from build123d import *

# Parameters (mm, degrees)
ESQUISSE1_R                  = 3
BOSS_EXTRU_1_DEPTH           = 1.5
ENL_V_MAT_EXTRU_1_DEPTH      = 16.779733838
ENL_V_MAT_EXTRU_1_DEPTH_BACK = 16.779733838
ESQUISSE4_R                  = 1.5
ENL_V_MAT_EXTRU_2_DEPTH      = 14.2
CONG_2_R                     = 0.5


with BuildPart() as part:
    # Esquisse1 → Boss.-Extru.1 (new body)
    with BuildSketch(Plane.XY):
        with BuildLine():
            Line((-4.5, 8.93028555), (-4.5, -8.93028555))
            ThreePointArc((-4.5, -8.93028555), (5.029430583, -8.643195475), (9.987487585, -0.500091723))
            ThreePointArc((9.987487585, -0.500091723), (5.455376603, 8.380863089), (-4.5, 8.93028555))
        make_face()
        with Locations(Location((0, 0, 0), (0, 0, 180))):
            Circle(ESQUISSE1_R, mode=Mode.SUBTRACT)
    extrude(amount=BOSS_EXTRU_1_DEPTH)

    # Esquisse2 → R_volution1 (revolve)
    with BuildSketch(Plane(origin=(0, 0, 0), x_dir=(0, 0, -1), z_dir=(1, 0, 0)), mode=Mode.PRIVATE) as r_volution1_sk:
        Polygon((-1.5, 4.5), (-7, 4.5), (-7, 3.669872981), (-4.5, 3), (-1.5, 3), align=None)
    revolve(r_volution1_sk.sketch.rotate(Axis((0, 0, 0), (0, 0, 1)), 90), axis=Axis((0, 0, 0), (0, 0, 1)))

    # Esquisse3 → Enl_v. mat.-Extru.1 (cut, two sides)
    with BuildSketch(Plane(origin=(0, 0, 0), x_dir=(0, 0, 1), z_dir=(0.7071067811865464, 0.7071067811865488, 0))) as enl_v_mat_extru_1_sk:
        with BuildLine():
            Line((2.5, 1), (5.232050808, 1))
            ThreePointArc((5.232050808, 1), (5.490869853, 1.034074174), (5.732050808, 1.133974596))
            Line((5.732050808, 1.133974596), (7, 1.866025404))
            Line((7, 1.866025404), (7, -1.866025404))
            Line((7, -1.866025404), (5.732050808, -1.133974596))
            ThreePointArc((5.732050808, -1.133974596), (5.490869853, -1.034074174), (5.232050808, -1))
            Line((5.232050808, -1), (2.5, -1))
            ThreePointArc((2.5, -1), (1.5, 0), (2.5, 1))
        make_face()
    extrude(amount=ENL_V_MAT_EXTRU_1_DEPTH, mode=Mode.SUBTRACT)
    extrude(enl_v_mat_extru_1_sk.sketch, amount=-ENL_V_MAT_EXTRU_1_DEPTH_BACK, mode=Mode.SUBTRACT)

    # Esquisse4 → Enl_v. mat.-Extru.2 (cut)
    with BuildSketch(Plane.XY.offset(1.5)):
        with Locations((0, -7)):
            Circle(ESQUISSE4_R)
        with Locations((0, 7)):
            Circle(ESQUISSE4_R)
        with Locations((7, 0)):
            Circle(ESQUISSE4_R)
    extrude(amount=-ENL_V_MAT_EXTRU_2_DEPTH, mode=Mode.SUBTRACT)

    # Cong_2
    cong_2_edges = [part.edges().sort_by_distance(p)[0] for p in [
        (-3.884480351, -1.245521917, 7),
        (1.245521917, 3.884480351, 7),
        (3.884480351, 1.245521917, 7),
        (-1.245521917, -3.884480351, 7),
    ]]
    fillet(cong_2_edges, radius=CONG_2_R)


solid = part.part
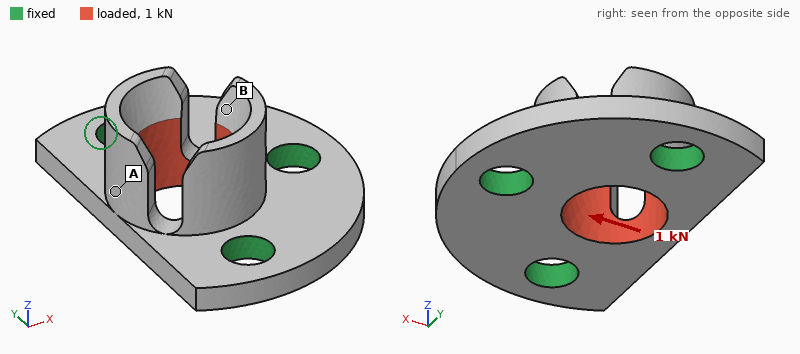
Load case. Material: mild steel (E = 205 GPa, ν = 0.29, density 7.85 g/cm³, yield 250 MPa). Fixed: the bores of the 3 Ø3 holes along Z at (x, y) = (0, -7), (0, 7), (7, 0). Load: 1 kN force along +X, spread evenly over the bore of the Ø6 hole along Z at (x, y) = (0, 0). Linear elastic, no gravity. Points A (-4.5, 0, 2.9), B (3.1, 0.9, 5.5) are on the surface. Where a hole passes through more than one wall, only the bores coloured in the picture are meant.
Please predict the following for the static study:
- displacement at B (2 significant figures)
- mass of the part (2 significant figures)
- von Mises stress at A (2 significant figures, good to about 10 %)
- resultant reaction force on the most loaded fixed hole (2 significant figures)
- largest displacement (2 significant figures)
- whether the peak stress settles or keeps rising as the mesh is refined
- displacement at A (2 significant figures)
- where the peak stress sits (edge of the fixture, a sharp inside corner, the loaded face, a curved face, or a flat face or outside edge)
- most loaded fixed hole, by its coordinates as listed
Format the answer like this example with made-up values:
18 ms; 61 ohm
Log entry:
4.4 µm; 3.4 g; 53 MPa; 410 N; 15 µm; keeps rising; 8.8 µm; edge of the fixture; (7, 0)
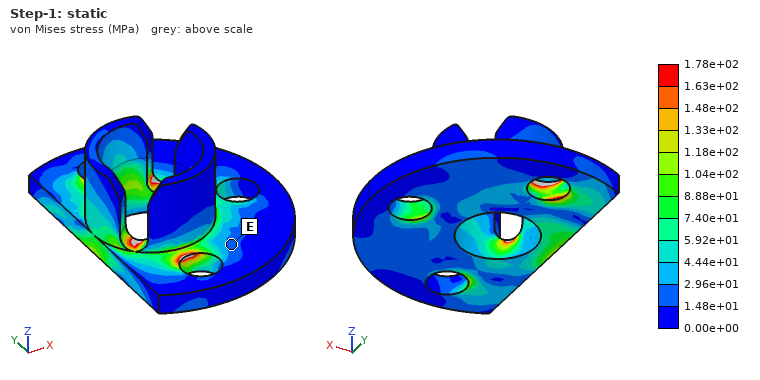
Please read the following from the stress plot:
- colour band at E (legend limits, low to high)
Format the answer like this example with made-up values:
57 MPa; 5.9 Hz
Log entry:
1.48e+01 to 2.96e+01 MPa
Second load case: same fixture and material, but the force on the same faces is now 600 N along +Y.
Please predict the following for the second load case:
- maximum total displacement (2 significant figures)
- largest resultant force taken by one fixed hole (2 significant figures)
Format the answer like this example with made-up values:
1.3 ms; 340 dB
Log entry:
3.5 µm; 260 N
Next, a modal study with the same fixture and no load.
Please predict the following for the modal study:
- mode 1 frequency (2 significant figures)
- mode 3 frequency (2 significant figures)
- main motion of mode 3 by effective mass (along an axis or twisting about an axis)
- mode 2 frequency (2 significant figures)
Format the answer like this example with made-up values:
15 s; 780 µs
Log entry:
29 kHz; 52 kHz; along Y; 37 kHz
